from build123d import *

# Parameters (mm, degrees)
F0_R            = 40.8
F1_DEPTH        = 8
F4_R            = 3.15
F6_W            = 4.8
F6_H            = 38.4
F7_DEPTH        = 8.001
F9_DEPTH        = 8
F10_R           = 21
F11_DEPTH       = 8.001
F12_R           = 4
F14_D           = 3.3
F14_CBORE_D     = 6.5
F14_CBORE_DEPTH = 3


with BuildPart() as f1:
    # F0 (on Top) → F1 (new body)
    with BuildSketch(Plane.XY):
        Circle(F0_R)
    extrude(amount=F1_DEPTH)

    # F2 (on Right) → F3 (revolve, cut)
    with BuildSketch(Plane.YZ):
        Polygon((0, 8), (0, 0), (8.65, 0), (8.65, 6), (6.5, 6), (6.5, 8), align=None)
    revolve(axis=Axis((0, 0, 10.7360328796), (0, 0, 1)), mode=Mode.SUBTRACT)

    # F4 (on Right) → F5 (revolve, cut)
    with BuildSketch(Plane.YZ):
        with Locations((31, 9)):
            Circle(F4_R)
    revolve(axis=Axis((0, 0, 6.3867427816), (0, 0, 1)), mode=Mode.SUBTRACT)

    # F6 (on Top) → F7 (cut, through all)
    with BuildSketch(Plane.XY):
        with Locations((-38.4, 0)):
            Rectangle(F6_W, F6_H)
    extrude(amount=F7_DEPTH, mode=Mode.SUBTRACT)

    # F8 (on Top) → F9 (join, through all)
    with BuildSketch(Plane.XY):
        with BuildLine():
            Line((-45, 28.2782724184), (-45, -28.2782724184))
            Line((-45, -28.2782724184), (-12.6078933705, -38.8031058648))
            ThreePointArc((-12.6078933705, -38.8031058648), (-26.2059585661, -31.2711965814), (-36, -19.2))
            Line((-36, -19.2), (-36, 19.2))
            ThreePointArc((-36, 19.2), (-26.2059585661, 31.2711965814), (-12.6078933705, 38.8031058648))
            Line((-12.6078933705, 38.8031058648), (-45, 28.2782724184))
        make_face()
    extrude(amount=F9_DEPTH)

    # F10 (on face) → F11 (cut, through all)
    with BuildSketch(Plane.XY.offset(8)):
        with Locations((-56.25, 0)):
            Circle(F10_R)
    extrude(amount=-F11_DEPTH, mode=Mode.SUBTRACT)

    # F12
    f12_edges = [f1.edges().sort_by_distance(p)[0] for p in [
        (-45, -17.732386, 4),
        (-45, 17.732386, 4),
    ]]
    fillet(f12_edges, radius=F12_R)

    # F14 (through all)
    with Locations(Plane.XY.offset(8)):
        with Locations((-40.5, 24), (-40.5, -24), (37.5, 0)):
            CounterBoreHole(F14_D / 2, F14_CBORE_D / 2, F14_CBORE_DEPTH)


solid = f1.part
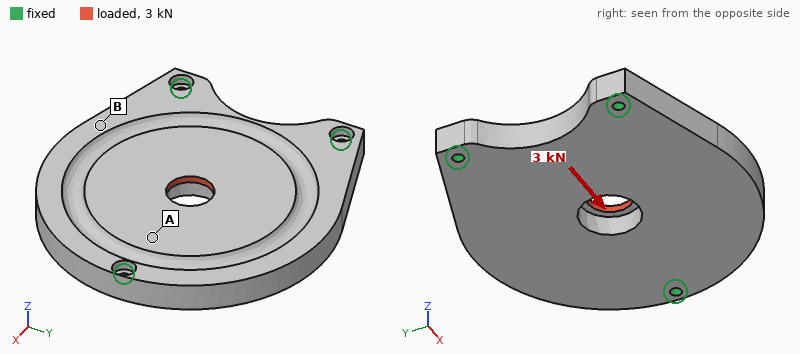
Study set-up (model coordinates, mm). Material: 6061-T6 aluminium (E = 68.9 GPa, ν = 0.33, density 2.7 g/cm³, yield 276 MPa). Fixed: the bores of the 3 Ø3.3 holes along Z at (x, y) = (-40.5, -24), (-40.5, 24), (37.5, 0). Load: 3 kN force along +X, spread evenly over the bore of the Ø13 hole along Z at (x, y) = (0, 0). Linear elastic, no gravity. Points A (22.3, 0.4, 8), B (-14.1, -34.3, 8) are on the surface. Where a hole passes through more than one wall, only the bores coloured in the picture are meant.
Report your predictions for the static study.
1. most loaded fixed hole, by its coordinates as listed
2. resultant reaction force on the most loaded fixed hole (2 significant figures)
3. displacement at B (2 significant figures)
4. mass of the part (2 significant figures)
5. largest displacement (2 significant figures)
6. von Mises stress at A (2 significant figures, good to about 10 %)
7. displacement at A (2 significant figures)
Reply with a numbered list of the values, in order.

1. (37.5, 0)
2. 1.2 kN
3. 2.4 µm
4. 110 g
5. 9.0 µm
6. 11 MPa
7. 3.3 µm
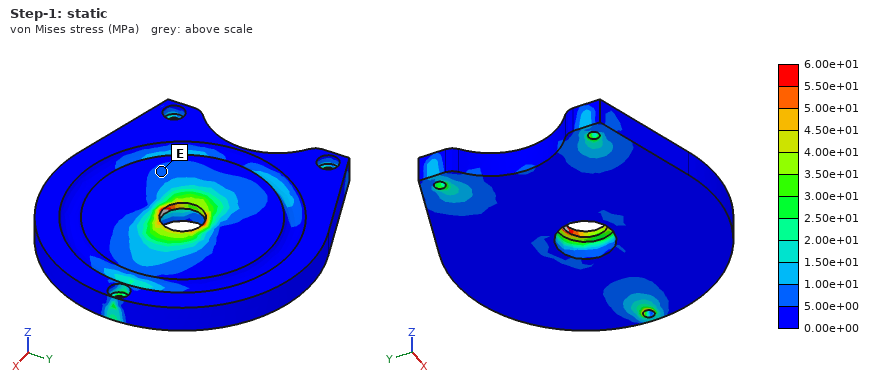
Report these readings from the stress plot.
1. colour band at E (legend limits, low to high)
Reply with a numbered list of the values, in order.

1. 5.00e+00 to 1.00e+01 MPa
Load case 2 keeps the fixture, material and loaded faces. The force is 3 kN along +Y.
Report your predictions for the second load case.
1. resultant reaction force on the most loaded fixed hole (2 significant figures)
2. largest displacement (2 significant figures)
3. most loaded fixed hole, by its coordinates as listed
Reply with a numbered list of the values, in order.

1. 1.3 kN
2. 34 µm
3. (37.5, 0)
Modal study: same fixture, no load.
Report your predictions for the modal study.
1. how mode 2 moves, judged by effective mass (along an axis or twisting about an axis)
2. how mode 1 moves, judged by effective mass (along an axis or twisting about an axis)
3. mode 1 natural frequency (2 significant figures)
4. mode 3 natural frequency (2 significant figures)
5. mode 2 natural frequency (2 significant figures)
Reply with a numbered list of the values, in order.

1. along Z
2. twisting about X
3. 3000 Hz
4. 7600 Hz
5. 3400 Hz
